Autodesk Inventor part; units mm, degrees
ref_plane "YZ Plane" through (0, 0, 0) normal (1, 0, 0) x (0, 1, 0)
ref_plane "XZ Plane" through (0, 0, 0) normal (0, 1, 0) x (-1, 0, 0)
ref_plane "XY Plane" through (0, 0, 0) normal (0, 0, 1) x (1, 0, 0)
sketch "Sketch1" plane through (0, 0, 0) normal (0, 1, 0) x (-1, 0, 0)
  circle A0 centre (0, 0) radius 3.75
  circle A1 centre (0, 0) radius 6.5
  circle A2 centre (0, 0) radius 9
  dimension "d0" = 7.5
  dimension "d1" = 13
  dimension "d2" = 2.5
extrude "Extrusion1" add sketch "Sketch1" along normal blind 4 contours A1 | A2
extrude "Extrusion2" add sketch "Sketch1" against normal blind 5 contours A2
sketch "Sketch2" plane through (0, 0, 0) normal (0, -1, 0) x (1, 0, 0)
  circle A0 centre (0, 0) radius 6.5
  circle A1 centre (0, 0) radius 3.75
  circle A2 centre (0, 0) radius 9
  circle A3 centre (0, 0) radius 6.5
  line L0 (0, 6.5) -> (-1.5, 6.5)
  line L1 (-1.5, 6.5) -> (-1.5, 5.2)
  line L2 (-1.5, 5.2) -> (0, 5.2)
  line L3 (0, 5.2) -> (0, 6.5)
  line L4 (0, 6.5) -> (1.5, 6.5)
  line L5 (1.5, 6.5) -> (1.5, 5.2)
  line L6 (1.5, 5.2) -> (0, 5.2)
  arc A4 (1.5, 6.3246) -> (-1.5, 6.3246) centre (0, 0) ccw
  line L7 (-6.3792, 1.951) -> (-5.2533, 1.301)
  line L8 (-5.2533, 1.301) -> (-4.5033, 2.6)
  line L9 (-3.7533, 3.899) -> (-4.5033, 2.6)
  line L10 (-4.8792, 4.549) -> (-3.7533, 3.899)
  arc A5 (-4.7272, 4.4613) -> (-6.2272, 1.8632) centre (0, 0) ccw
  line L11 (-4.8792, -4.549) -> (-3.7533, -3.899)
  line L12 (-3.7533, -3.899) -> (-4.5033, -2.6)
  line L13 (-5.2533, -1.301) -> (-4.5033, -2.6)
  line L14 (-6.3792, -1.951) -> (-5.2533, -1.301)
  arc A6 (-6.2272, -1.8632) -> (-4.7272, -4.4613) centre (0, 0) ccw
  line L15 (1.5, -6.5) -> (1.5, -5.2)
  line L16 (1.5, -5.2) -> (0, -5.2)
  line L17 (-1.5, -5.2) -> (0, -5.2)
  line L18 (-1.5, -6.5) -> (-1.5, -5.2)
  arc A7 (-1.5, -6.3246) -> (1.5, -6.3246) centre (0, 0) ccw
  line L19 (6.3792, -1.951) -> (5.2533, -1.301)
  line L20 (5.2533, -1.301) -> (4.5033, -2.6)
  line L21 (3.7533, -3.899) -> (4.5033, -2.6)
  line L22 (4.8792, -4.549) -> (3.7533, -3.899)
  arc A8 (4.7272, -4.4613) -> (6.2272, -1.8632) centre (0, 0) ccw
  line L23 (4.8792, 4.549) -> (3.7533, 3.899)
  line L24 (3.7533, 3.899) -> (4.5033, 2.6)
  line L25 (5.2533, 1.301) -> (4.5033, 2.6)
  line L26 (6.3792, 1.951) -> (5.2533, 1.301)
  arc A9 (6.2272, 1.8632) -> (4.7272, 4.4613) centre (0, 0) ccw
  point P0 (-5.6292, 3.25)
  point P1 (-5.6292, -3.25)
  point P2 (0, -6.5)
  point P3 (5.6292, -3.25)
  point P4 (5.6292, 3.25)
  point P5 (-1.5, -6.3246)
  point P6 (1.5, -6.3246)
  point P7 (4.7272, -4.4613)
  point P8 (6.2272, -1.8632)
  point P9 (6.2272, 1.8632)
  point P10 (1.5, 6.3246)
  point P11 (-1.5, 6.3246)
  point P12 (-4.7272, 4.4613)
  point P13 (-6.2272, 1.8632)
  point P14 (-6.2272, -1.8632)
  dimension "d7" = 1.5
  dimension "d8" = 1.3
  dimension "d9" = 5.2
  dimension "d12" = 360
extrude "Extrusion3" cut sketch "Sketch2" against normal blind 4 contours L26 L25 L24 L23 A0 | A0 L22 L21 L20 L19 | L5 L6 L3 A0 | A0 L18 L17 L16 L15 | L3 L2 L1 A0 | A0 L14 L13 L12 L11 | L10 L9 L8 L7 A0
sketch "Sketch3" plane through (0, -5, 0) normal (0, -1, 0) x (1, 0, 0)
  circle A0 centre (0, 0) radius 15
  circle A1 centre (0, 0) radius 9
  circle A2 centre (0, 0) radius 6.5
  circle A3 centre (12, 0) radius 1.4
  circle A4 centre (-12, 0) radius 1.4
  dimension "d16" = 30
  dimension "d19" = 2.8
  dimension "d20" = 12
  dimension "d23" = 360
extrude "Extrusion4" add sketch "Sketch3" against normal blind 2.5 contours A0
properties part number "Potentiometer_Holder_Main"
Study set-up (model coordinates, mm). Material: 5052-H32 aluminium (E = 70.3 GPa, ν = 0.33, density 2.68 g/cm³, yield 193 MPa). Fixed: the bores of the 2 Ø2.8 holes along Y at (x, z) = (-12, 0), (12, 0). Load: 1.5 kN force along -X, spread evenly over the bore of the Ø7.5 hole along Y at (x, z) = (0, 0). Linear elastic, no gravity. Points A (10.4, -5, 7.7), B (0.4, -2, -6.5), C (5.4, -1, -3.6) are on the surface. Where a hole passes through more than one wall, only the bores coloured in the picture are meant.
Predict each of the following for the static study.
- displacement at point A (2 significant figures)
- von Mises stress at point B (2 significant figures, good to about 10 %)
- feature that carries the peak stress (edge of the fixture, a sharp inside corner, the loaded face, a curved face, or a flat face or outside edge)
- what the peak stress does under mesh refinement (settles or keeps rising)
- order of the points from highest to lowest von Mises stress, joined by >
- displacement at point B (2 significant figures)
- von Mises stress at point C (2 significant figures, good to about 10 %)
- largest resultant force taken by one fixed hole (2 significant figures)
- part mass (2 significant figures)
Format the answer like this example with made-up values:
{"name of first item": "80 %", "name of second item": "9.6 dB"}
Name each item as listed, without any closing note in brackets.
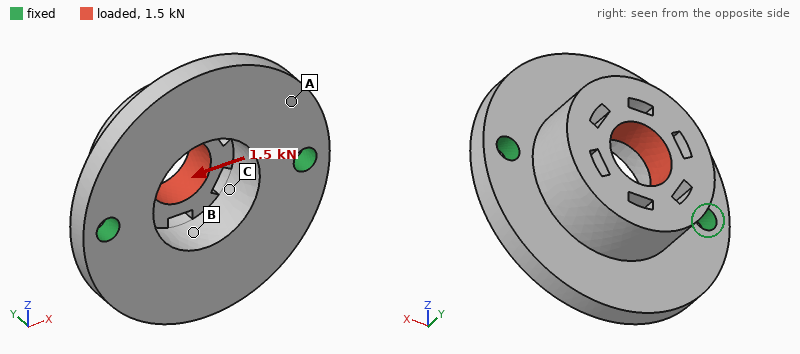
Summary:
{"displacement at point A": "5.3 µm", "von Mises stress at point B": "25 MPa", "feature that carries the peak stress": "edge of the fixture", "what the peak stress does under mesh refinement": "keeps rising", "order of the points from highest to lowest von Mises stress, joined by >": "C > B > A", "displacement at point B": "5.7 µm", "von Mises stress at point C": "35 MPa", "largest resultant force taken by one fixed hole": "860 N", "part mass": "6.6 g"}
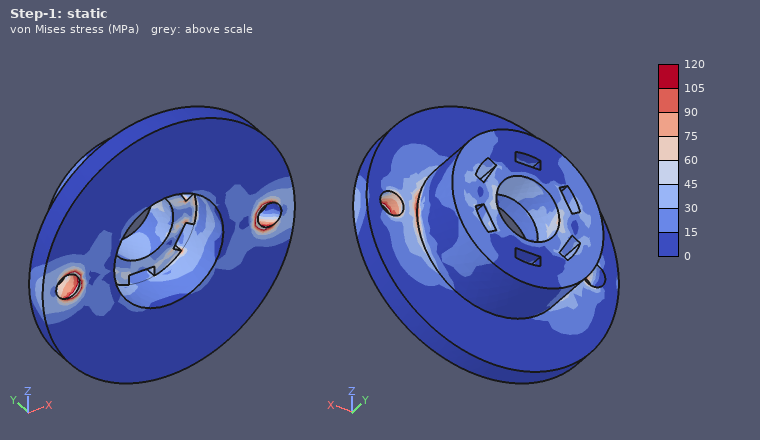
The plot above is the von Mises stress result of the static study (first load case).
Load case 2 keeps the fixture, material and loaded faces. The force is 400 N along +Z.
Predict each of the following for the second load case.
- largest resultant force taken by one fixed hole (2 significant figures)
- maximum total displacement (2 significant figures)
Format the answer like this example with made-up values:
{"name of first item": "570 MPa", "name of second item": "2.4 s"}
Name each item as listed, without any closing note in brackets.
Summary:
{"largest resultant force taken by one fixed hole": "200 N", "maximum total displacement": "35 µm"}
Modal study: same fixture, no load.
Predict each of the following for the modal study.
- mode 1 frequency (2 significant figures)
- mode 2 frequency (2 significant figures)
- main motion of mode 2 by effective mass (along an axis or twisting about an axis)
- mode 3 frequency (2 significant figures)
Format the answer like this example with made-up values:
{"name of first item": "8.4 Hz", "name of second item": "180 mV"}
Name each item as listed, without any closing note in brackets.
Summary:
{"mode 1 frequency": "8000 Hz", "mode 2 frequency": "18 kHz", "main motion of mode 2 by effective mass": "along Y", "mode 3 frequency": "30 kHz"}
